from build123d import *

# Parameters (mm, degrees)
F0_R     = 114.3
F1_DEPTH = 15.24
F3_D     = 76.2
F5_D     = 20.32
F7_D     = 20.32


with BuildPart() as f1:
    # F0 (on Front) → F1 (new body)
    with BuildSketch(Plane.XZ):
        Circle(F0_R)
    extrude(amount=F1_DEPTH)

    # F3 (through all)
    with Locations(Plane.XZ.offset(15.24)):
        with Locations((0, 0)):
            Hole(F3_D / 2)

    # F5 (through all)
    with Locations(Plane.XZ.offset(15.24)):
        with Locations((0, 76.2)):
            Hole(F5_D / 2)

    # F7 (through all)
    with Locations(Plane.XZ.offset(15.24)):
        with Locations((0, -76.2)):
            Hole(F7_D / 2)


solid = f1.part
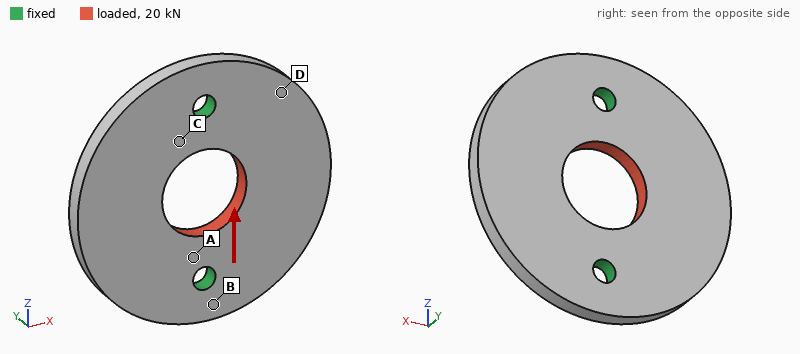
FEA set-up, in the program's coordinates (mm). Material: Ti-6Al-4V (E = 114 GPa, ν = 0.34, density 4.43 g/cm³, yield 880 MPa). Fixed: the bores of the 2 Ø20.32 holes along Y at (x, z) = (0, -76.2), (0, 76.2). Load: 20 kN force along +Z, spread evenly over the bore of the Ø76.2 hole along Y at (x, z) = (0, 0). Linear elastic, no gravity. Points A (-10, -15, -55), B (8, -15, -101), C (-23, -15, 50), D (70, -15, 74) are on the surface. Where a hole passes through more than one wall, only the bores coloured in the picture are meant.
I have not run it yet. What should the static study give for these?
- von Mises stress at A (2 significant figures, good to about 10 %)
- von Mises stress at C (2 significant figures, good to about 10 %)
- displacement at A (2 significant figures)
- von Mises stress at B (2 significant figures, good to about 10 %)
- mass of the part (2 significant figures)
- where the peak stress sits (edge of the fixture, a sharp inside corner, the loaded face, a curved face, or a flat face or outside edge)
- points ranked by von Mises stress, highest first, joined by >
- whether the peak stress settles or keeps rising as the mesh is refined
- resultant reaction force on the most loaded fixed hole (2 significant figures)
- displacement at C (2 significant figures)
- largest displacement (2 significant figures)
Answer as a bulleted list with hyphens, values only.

- 11 MPa
- 9.0 MPa
- 1.7 µm
- 4.2 MPa
- 2.4 kg
- edge of the fixture
- A > C > B > D
- keeps rising
- 10 kN
- 3.2 µm
- 6.5 µm
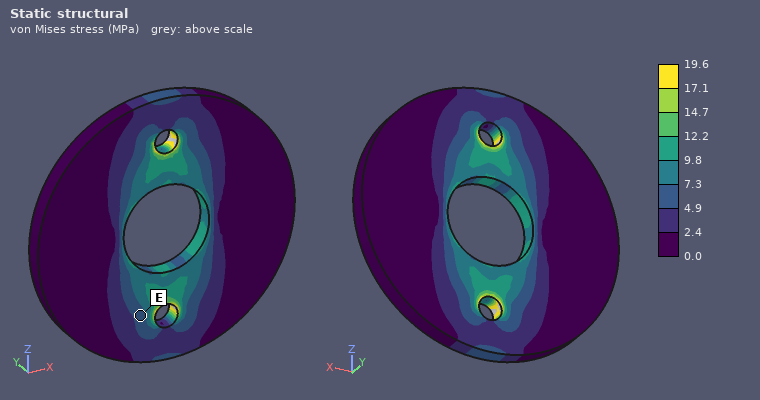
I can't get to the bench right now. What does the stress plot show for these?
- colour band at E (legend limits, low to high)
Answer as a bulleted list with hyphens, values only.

- 4.9 to 7.3 MPa
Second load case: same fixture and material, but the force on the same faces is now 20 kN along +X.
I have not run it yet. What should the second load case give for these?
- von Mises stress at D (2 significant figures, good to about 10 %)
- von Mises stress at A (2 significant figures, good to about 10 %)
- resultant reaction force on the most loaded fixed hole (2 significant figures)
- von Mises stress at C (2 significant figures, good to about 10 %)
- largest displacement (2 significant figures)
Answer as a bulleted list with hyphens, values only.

- 2.9 MPa
- 10 MPa
- 10 kN
- 8.5 MPa
- 7.3 µm
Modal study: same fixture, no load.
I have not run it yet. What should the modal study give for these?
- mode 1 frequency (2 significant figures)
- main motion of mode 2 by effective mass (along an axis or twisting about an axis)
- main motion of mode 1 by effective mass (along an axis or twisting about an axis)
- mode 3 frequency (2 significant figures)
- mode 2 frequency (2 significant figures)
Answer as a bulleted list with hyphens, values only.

- 1000 Hz
- along Y
- twisting about Z
- 2500 Hz
- 1100 Hz
